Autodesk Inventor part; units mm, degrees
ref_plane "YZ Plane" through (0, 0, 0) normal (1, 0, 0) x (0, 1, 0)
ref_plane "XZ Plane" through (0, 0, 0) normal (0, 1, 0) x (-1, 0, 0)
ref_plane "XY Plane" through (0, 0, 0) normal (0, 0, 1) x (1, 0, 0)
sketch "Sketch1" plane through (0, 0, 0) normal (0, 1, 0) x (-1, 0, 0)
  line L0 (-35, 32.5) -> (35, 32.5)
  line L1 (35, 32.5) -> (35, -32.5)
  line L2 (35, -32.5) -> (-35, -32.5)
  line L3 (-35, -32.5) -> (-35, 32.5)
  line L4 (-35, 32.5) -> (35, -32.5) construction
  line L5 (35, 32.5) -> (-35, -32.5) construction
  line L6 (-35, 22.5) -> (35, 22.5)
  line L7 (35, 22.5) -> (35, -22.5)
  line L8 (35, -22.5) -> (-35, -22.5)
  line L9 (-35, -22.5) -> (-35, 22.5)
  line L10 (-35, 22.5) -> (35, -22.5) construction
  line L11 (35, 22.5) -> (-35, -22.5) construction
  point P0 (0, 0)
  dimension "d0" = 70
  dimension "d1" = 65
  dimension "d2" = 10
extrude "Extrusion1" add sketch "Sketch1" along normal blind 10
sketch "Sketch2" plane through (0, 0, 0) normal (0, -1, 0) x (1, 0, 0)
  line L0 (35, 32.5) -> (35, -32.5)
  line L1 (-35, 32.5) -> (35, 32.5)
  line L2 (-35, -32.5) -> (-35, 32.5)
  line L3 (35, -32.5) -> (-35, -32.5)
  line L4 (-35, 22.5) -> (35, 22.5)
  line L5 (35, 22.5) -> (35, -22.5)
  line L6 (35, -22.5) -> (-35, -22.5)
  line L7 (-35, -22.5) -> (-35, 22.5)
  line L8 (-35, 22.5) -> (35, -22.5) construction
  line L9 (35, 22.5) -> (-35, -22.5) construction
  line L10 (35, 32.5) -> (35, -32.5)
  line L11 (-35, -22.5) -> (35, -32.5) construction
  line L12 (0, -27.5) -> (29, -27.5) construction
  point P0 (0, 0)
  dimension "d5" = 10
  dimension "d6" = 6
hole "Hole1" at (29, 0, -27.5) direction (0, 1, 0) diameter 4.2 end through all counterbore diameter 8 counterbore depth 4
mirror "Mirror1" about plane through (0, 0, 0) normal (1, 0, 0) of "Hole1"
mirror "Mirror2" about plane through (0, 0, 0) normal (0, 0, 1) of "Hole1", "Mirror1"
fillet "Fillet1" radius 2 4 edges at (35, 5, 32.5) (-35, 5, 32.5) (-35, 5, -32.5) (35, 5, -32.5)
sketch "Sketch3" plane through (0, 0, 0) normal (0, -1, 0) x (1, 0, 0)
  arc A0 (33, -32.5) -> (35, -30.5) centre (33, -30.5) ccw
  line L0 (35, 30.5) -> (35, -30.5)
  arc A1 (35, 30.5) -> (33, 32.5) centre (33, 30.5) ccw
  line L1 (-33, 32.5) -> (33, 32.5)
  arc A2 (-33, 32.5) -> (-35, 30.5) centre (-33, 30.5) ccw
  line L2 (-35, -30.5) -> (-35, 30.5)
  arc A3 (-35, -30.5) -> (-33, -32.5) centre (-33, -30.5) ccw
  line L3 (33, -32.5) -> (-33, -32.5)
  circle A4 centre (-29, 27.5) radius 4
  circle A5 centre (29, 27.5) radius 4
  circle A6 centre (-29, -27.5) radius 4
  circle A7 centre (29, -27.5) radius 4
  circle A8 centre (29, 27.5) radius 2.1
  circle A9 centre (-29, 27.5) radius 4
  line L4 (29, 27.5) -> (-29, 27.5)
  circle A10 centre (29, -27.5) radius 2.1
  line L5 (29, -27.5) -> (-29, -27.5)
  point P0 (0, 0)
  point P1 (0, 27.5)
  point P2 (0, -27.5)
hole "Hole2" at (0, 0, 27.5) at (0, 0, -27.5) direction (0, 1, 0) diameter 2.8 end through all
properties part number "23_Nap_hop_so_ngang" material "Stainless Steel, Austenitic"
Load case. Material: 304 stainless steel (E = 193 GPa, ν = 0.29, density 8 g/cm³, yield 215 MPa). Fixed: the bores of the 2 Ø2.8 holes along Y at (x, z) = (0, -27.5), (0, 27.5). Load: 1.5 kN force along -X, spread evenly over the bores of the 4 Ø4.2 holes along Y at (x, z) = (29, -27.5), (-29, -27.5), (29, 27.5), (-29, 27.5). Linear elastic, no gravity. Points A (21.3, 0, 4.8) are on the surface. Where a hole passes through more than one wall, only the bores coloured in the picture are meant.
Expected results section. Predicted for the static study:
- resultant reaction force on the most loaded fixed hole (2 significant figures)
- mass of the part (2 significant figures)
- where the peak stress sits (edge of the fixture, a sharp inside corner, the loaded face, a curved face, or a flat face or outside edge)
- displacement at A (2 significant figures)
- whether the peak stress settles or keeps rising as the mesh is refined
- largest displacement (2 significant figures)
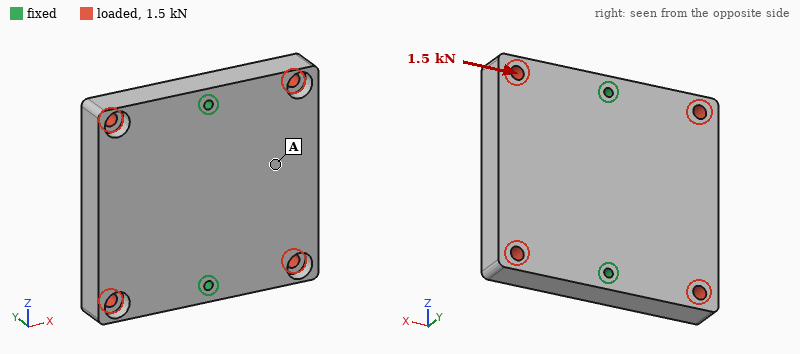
750 N
350 g
edge of the fixture
1.0 µm
keeps rising
2.2 µm
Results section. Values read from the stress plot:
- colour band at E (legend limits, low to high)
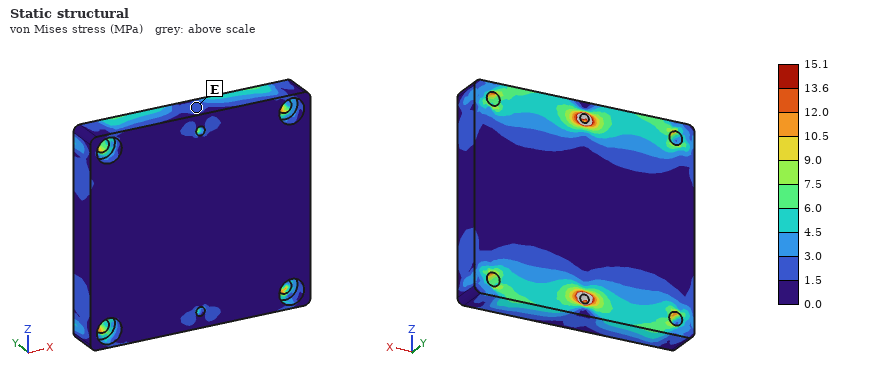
1.5 to 3.0 MPa
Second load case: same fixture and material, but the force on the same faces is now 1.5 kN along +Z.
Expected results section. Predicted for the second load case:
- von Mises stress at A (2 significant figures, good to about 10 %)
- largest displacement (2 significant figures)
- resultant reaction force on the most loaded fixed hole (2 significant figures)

2.2 MPa
1.5 µm
750 N
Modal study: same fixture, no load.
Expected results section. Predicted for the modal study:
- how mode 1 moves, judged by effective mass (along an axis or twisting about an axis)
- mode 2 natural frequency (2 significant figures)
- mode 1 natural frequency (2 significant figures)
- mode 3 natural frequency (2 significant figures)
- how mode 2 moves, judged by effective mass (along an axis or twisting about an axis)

twisting about Z
5400 Hz
3500 Hz
8700 Hz
along Y
